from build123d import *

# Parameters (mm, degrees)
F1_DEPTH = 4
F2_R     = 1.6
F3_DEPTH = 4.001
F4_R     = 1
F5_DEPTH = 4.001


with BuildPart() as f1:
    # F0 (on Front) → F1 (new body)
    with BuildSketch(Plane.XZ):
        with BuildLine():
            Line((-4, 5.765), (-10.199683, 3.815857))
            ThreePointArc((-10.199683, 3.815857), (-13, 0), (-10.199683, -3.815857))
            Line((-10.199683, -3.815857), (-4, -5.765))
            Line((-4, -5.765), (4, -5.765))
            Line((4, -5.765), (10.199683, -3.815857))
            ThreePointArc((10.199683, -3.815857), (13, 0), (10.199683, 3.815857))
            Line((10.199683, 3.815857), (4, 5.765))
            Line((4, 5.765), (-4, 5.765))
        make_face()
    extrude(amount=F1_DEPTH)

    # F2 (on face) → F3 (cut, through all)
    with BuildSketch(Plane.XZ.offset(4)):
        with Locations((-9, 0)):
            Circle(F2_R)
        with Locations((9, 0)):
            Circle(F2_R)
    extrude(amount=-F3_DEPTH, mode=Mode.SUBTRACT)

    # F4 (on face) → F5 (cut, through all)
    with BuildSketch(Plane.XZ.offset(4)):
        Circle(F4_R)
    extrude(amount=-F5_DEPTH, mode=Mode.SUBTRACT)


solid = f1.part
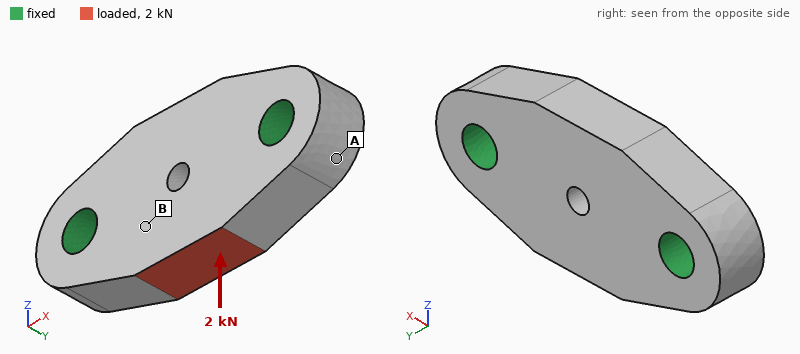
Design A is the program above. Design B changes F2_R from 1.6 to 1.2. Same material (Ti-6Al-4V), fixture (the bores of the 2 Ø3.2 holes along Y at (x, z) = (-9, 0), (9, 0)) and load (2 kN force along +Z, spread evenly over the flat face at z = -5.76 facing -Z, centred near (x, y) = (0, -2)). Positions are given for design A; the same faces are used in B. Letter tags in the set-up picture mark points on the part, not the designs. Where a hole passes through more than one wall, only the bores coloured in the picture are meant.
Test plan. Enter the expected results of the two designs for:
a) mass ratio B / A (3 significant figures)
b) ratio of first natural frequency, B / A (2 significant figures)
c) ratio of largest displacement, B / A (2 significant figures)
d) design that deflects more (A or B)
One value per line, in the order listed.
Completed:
1.03
0.90
1.1
B
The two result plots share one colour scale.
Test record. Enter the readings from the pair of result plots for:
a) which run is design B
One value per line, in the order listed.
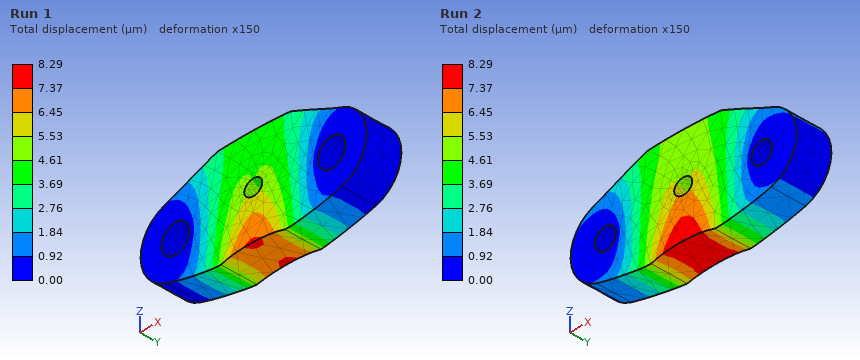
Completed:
Run 2
